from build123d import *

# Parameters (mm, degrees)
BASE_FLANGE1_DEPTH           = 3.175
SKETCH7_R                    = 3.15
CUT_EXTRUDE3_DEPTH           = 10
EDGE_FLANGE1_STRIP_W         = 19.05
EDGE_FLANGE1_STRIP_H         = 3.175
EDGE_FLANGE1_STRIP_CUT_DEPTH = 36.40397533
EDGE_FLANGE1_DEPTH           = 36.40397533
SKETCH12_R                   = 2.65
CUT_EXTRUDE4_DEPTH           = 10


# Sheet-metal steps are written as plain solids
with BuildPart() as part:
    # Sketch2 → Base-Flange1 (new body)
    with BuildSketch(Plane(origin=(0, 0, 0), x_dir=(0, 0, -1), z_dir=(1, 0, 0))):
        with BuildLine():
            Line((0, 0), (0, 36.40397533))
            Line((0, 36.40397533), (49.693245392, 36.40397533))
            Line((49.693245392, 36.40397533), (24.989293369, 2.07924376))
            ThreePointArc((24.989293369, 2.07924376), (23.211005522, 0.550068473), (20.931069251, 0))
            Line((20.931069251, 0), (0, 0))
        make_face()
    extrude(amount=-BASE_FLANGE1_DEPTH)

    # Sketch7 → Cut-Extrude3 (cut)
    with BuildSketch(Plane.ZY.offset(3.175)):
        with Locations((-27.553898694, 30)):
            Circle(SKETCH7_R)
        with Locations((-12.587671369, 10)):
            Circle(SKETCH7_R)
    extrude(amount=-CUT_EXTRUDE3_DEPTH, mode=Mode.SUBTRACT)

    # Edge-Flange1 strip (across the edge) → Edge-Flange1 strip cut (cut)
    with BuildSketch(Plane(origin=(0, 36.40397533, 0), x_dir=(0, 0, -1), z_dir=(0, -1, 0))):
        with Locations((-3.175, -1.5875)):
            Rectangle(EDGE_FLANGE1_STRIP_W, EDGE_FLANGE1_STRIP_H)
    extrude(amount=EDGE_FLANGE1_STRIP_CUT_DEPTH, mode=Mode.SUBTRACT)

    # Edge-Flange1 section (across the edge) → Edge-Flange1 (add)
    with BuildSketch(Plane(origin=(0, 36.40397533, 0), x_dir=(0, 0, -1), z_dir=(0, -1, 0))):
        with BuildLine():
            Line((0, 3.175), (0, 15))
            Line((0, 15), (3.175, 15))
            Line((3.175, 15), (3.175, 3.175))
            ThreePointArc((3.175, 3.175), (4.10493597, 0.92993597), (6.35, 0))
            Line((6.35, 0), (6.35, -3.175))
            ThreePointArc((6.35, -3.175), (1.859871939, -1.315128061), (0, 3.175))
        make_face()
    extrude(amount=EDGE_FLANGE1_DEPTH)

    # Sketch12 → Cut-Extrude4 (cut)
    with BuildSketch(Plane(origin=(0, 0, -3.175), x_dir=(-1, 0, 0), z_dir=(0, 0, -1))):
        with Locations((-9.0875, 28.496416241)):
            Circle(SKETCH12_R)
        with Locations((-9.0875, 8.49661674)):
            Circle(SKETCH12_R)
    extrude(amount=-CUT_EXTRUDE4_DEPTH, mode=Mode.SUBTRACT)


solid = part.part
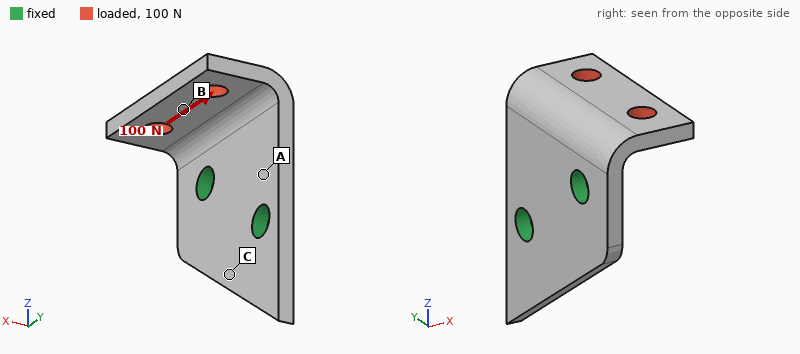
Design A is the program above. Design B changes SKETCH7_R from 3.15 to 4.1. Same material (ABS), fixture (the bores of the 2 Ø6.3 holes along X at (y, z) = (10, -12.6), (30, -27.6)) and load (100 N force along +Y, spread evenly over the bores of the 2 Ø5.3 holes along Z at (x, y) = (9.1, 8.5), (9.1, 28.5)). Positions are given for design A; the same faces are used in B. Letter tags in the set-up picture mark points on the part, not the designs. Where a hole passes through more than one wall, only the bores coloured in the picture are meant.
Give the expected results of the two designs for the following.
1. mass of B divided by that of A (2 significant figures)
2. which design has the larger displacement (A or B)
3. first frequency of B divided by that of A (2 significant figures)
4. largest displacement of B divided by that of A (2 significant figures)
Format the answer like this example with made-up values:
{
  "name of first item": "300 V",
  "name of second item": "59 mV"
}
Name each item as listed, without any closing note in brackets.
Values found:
{
  "mass of B divided by that of A": "0.97",
  "which design has the larger displacement": "A",
  "first frequency of B divided by that of A": "1.1",
  "largest displacement of B divided by that of A": "0.84"
}
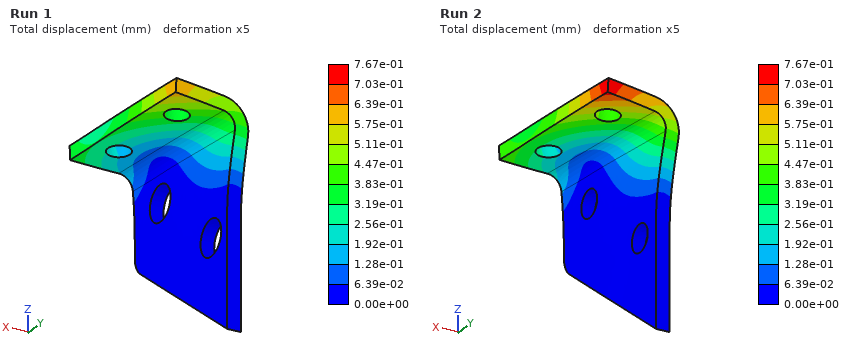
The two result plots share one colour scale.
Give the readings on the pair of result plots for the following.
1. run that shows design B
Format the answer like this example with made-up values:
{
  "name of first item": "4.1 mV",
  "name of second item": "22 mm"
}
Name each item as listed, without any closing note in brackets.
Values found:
{
  "run that shows design B": "Run 1"
}
